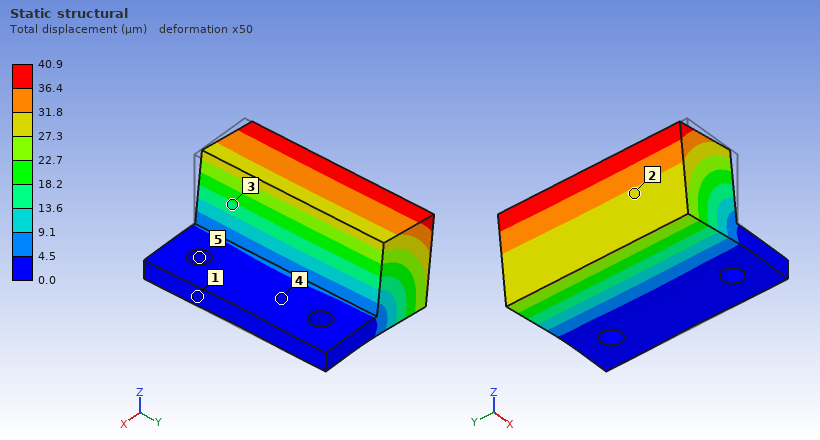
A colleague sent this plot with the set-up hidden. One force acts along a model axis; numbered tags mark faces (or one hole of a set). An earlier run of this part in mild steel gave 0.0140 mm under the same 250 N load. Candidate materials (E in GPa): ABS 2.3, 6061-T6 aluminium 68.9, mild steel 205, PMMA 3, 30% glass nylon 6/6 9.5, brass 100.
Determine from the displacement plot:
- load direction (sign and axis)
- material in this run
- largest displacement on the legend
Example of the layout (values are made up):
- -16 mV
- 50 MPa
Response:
- -X
- 6061-T6 aluminium
- 40.9 µm
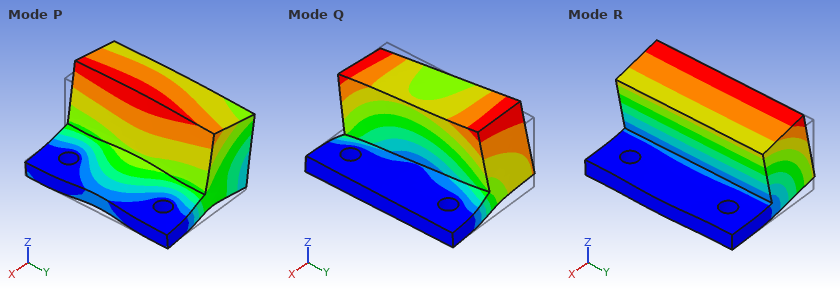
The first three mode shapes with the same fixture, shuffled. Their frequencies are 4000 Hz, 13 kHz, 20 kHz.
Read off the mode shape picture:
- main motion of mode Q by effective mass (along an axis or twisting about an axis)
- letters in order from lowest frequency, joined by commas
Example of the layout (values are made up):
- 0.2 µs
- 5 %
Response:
- along Y
- R, Q, P
